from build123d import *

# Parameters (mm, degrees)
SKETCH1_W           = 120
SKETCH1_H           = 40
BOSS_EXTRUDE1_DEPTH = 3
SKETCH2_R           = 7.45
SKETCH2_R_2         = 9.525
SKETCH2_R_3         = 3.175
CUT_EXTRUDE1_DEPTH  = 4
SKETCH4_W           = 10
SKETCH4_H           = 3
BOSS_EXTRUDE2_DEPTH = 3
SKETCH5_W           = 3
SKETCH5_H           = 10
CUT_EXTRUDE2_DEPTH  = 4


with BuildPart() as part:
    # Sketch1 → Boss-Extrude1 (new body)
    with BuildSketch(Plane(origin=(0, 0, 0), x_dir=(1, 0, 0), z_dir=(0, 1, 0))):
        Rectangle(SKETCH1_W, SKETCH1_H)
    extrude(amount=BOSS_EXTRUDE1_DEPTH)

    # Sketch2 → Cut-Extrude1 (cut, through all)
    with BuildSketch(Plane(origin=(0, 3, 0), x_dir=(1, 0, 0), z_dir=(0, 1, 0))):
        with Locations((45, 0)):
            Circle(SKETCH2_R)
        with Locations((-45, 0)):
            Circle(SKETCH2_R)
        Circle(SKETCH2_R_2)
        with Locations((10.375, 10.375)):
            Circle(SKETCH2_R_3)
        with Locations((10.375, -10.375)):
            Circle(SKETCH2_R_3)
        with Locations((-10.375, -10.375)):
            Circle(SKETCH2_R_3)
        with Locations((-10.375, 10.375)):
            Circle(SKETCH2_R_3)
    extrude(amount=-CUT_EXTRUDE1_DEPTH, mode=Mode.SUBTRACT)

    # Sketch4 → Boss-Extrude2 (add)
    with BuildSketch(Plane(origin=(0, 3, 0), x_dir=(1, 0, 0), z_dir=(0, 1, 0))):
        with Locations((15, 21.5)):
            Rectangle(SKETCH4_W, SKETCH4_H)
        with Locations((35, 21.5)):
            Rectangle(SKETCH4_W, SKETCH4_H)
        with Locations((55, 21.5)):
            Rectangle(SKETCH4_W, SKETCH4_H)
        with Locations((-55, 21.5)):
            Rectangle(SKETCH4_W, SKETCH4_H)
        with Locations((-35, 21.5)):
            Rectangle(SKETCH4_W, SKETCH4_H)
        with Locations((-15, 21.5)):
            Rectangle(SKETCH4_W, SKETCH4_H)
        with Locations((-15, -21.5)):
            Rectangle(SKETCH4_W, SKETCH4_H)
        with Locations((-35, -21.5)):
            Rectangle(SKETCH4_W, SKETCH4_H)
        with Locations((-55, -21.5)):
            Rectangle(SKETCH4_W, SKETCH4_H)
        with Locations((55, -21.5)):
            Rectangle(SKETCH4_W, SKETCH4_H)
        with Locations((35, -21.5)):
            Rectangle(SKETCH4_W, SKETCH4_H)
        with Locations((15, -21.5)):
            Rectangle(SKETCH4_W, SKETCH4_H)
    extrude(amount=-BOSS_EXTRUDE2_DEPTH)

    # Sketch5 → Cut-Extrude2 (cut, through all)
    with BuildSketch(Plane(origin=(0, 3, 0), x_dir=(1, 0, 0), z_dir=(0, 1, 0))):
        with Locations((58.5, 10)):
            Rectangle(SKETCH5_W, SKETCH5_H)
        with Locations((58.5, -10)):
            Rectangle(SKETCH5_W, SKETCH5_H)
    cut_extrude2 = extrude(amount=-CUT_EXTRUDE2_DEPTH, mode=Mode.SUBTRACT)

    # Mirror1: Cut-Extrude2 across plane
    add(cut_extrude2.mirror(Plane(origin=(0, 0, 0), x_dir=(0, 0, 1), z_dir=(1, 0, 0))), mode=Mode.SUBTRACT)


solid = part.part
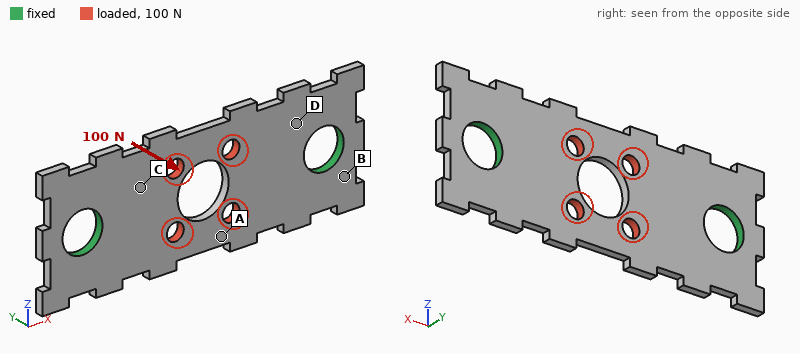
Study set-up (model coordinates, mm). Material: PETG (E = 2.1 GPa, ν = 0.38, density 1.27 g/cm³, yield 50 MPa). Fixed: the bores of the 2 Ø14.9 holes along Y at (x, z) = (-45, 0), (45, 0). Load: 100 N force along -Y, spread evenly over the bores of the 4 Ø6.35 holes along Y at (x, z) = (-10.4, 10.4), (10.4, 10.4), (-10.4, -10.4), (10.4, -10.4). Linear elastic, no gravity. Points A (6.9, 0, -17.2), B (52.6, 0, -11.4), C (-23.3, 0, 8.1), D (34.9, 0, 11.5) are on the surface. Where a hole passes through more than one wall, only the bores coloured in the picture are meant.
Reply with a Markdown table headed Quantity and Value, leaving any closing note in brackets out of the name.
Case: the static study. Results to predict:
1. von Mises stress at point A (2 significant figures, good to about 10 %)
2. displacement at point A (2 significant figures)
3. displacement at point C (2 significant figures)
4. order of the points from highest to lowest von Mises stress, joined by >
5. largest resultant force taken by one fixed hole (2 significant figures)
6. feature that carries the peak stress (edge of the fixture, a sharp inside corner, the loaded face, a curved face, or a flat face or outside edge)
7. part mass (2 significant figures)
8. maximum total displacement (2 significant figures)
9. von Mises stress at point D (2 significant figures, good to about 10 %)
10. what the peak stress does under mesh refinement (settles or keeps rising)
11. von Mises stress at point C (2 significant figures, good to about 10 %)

| Quantity | Value |
|---|---|
| von Mises stress at point A | 12 MPa |
| displacement at point A | 1.4 mm |
| displacement at point C | 0.56 mm |
| order of the points from highest to lowest von Mises stress, joined by > | A > D > C > B |
| largest resultant force taken by one fixed hole | 50 N |
| feature that carries the peak stress | edge of the fixture |
| part mass | 16 g |
| maximum total displacement | 1.5 mm |
| von Mises stress at point D | 9.7 MPa |
| what the peak stress does under mesh refinement | keeps rising |
| von Mises stress at point C | 4.3 MPa |
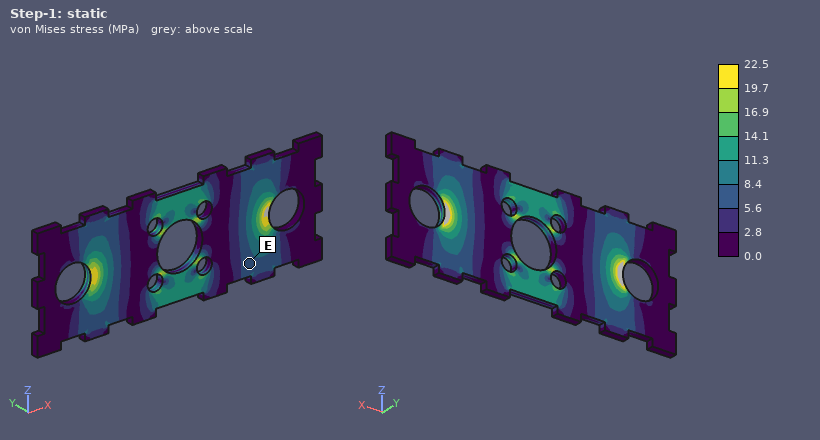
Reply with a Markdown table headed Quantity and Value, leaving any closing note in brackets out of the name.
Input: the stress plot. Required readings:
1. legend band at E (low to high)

| Quantity | Value |
|---|---|
| legend band at E | 5.6 to 8.4 MPa |
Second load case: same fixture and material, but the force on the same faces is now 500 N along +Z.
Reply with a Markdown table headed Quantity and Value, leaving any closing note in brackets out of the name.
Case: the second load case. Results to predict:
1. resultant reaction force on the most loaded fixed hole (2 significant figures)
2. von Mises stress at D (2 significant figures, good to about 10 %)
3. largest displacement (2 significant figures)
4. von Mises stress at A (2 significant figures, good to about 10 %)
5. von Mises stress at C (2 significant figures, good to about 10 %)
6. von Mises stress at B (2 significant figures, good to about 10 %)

| Quantity | Value |
|---|---|
| resultant reaction force on the most loaded fixed hole | 250 N |
| von Mises stress at D | 3.3 MPa |
| largest displacement | 0.20 mm |
| von Mises stress at A | 6.3 MPa |
| von Mises stress at C | 4.4 MPa |
| von Mises stress at B | 1.8 MPa |
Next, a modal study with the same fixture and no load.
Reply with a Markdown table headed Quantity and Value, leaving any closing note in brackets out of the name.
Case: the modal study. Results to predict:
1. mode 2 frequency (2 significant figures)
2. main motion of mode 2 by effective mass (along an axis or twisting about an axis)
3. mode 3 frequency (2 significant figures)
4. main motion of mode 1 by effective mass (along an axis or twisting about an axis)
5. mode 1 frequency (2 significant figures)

| Quantity | Value |
|---|---|
| mode 2 frequency | 780 Hz |
| main motion of mode 2 by effective mass | twisting about X |
| mode 3 frequency | 1400 Hz |
| main motion of mode 1 by effective mass | along Y |
| mode 1 frequency | 630 Hz |
